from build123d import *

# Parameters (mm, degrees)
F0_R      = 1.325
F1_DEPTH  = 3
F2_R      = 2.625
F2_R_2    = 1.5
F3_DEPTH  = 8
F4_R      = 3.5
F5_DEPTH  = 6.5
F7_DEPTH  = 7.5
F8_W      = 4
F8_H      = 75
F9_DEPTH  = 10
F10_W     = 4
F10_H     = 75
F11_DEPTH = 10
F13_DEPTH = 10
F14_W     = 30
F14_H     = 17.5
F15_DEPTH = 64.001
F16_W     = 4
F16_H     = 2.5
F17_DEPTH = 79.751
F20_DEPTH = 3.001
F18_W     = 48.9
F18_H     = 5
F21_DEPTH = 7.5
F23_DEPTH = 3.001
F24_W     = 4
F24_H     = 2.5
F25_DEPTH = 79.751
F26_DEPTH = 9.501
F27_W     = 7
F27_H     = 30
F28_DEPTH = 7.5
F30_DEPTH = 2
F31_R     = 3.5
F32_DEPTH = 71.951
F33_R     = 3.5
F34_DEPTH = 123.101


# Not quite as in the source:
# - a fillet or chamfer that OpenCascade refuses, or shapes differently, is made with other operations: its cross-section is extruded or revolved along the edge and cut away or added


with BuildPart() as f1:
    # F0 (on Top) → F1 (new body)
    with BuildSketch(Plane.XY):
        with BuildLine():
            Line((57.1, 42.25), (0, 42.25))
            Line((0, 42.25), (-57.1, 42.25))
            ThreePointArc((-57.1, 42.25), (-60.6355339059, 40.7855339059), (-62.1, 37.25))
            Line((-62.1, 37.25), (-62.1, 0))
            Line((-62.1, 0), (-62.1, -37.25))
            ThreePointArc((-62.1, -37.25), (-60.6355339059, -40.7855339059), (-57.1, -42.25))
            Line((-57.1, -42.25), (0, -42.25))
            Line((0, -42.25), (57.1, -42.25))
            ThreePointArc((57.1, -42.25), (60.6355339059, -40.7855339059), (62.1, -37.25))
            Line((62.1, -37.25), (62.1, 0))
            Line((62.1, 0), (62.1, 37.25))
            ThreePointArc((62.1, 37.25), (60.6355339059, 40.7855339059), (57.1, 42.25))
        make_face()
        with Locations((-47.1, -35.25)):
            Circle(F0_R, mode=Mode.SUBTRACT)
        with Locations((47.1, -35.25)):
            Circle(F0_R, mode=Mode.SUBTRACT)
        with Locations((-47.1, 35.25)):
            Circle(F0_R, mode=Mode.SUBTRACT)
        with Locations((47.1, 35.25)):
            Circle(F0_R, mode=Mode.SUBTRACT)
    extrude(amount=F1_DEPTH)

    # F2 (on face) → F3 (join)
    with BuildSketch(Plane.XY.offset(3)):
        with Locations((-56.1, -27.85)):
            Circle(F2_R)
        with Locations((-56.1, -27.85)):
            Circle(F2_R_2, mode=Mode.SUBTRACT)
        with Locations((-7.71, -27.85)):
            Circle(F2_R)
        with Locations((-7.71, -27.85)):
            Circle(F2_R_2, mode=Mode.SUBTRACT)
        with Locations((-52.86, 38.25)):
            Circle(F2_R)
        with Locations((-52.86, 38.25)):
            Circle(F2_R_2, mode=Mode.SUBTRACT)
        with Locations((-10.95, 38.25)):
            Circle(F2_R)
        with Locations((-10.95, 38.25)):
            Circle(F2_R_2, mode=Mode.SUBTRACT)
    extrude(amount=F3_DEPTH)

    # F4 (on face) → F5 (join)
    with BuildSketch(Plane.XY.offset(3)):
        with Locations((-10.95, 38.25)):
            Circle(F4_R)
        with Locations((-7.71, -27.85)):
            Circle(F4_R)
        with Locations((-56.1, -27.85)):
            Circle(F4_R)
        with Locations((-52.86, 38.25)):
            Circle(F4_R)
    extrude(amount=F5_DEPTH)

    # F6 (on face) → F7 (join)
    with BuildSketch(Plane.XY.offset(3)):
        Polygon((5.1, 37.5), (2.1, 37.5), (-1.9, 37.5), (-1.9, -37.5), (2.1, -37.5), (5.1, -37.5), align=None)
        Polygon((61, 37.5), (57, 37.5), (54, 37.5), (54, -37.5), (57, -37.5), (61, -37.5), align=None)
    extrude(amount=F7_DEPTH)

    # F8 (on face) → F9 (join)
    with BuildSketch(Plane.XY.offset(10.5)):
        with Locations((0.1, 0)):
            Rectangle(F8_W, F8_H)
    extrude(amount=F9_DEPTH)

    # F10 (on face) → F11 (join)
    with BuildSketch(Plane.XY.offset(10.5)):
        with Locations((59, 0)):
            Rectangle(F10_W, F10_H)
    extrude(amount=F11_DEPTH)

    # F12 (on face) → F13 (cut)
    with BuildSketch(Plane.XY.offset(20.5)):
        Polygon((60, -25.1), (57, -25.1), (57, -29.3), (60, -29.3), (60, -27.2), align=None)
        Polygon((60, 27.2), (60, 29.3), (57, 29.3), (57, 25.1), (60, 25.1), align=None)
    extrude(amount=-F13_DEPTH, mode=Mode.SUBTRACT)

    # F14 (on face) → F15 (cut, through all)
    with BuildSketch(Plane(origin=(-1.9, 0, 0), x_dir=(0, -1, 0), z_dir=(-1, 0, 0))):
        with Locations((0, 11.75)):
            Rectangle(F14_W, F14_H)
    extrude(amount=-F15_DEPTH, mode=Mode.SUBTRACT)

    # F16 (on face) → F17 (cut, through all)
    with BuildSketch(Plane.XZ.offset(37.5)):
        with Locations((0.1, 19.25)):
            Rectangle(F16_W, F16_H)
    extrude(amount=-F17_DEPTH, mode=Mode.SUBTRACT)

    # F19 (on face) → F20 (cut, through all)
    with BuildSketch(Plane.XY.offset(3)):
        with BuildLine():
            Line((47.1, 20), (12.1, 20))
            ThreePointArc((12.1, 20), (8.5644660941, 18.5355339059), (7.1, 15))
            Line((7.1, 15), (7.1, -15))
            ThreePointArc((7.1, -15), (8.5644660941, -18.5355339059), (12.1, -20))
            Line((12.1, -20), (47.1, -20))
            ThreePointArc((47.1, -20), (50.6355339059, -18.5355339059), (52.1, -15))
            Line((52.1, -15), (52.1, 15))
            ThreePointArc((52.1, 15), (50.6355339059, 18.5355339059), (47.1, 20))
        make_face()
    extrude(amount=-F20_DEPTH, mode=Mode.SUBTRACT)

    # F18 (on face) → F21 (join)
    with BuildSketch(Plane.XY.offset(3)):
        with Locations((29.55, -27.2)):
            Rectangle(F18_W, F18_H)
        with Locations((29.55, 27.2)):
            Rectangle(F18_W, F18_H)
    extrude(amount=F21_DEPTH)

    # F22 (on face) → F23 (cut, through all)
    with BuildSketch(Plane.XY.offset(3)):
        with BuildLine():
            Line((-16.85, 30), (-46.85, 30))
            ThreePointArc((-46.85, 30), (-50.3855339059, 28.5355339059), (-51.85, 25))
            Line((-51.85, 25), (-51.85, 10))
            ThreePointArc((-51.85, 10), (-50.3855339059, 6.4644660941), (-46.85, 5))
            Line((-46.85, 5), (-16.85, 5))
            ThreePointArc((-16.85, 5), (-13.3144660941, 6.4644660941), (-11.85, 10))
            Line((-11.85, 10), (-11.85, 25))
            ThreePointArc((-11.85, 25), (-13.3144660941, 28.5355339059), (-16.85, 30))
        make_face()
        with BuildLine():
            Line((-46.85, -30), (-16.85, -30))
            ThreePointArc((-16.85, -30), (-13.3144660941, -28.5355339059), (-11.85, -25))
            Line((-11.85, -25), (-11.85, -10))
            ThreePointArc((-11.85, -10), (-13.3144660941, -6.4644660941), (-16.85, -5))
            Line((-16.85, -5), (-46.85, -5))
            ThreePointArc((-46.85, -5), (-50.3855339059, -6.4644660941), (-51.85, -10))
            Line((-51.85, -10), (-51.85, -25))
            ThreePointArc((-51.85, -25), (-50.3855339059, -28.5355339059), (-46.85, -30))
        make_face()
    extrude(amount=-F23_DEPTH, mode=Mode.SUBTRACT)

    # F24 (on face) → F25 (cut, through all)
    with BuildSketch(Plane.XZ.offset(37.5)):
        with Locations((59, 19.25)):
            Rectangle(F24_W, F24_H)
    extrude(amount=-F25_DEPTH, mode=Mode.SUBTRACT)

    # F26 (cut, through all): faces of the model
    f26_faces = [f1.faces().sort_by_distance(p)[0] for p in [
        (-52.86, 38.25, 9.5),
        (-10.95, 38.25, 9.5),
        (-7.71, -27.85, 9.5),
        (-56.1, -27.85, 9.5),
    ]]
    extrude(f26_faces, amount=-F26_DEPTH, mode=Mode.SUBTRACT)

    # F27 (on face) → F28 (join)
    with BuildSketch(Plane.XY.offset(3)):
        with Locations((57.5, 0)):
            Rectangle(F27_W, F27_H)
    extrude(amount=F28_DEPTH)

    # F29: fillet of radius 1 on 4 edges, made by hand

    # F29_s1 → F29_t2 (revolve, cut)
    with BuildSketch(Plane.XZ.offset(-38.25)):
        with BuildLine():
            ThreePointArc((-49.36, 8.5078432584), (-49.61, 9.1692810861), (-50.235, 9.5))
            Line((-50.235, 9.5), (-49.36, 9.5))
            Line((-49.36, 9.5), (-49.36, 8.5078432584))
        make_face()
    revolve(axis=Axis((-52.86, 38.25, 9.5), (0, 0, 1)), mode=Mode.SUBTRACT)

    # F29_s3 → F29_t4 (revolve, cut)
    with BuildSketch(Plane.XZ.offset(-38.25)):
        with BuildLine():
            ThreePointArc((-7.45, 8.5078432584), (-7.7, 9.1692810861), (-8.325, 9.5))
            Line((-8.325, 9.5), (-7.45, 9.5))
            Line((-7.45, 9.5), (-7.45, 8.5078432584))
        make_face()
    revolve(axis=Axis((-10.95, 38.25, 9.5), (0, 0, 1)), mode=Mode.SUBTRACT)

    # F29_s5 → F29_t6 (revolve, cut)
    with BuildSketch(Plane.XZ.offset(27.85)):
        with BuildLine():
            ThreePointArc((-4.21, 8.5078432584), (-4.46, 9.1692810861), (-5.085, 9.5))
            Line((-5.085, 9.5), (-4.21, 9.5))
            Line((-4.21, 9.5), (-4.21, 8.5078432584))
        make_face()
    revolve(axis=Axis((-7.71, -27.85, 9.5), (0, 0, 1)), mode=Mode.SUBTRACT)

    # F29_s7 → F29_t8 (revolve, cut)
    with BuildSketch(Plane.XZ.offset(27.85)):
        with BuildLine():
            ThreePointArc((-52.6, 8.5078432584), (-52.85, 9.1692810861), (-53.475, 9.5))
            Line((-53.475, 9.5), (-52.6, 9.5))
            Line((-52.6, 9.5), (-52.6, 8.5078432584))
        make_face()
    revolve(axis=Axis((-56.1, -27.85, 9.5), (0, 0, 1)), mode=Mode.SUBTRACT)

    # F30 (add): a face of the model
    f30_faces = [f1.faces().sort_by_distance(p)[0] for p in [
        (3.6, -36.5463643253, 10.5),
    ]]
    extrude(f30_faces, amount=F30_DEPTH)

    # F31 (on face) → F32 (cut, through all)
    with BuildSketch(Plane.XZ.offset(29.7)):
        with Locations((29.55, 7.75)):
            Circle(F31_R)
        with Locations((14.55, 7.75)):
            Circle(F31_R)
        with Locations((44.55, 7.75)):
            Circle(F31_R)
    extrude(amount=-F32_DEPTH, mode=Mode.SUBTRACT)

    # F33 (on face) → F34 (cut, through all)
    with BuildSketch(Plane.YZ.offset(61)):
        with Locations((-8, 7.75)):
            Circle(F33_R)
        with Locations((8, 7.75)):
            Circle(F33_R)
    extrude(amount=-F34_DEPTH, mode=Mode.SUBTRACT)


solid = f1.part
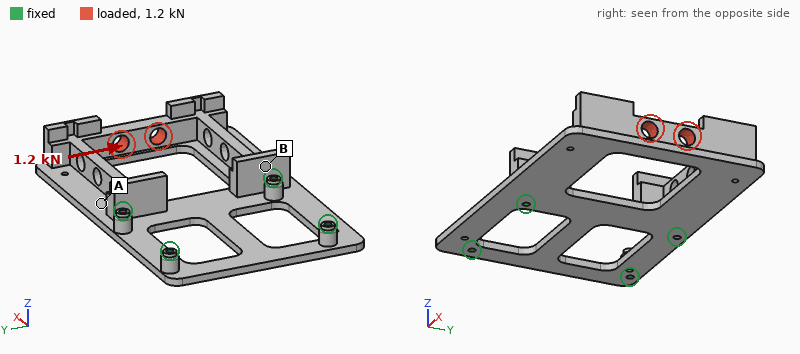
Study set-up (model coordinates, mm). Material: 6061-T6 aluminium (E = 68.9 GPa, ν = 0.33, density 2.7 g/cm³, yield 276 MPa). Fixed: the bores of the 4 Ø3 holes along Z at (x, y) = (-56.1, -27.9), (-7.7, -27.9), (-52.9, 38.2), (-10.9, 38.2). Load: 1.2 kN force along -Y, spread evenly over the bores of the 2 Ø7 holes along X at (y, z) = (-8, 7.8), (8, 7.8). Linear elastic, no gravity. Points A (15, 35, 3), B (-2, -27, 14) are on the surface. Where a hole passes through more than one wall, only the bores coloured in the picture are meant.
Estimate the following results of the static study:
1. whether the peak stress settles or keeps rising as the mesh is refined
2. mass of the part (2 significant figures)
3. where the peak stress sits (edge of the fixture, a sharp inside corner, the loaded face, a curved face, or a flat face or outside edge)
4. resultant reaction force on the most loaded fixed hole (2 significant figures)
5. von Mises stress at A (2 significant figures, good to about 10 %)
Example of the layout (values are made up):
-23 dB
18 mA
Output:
keeps rising
91 g
edge of the fixture
1.2 kN
39 MPa
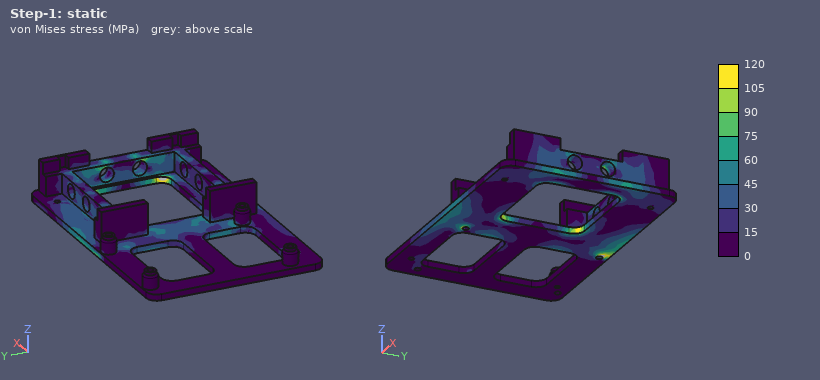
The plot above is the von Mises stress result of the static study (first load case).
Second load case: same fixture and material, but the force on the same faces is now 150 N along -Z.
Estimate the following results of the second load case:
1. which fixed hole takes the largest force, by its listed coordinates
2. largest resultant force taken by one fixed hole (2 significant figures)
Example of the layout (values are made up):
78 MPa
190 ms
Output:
(-7.7, -27.9)
140 N
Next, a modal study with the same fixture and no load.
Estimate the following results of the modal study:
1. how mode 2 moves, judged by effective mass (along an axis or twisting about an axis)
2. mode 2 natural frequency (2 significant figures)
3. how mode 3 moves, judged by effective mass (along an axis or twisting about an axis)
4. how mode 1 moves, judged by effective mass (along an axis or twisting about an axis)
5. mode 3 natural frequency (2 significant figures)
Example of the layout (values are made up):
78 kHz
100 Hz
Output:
twisting about X
1100 Hz
along Y
along Z
2600 Hz
